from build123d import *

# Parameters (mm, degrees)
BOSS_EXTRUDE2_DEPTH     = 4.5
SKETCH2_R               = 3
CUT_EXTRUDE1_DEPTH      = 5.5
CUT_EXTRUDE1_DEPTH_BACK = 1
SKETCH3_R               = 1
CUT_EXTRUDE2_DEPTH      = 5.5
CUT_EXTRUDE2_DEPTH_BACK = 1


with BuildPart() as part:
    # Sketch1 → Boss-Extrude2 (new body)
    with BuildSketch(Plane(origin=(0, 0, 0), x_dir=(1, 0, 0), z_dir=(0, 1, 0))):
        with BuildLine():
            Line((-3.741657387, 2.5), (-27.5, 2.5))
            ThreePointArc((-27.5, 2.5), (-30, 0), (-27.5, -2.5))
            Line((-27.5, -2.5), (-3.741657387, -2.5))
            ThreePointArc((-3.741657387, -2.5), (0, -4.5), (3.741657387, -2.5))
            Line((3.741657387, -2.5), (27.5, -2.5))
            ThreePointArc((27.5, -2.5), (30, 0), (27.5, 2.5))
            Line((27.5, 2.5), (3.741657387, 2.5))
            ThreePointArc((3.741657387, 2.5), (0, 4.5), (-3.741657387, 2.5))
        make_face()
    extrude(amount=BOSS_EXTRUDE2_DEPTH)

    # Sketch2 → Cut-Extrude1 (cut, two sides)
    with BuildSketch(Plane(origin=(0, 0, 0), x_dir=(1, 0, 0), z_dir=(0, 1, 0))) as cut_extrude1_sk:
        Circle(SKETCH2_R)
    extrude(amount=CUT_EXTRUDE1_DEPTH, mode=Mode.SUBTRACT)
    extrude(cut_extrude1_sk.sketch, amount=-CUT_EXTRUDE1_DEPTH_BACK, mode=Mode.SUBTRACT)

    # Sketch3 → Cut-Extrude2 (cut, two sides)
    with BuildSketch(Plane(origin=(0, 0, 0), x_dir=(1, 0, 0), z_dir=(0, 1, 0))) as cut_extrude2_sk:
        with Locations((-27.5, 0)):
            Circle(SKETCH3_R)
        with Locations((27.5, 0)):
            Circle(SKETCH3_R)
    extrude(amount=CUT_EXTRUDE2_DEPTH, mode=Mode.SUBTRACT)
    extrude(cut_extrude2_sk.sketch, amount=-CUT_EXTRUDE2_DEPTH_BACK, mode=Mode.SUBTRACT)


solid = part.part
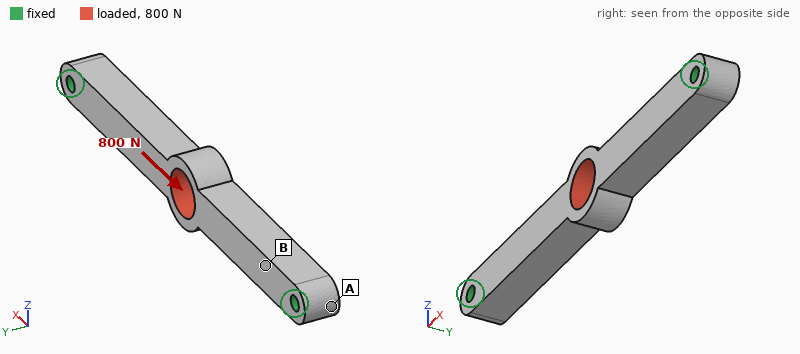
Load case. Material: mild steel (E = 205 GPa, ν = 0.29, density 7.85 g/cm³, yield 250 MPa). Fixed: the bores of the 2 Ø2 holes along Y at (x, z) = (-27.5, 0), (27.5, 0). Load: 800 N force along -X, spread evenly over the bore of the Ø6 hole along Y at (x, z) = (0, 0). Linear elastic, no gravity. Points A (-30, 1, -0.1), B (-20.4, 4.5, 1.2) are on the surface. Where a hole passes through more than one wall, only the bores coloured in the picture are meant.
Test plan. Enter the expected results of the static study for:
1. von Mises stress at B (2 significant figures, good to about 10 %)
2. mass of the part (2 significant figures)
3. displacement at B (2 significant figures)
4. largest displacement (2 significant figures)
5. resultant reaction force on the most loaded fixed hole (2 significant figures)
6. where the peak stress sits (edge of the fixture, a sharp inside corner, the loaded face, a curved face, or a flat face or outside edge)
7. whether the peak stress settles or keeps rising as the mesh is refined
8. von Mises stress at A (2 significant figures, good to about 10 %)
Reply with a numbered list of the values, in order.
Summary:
1. 18 MPa
2. 9.9 g
3. 0.61 µm
4. 2.6 µm
5. 400 N
6. edge of the fixture
7. keeps rising
8. 3.9 MPa
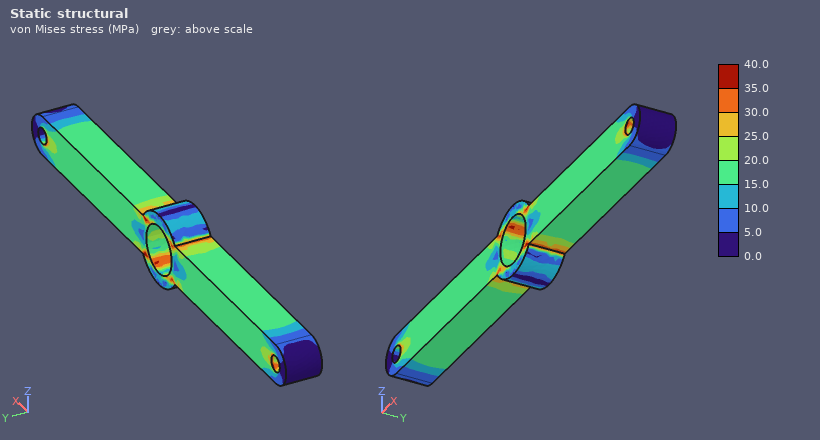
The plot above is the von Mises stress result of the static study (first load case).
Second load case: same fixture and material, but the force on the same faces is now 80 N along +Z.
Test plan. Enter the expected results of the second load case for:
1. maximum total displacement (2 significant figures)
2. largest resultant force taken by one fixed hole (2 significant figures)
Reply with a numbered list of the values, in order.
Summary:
1. 8.8 µm
2. 40 N
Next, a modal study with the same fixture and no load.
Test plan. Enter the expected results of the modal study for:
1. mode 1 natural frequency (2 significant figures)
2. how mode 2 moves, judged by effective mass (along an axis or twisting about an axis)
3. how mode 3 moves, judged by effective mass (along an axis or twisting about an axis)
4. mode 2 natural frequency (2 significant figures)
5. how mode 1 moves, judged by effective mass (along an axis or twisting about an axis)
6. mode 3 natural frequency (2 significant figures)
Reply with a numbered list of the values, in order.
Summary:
1. 6800 Hz
2. along Z
3. twisting about Y
4. 7800 Hz
5. along Y
6. 17 kHz
